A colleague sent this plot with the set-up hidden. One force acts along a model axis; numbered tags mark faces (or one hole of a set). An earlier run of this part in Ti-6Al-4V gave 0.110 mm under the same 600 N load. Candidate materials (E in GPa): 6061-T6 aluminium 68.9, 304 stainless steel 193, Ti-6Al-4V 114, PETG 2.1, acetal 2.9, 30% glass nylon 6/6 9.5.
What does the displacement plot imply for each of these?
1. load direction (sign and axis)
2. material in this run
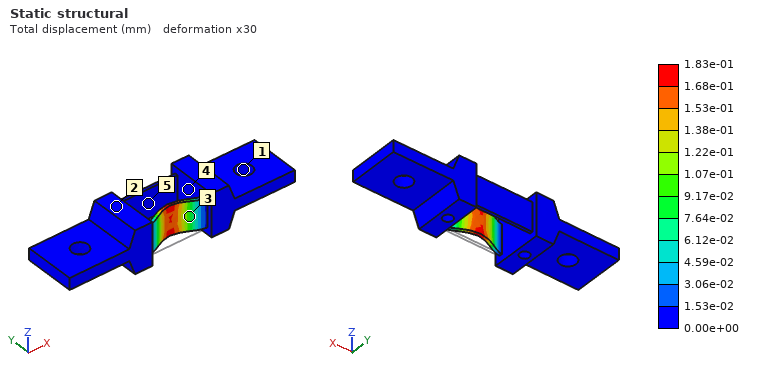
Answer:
+Y
6061-T6 aluminium
